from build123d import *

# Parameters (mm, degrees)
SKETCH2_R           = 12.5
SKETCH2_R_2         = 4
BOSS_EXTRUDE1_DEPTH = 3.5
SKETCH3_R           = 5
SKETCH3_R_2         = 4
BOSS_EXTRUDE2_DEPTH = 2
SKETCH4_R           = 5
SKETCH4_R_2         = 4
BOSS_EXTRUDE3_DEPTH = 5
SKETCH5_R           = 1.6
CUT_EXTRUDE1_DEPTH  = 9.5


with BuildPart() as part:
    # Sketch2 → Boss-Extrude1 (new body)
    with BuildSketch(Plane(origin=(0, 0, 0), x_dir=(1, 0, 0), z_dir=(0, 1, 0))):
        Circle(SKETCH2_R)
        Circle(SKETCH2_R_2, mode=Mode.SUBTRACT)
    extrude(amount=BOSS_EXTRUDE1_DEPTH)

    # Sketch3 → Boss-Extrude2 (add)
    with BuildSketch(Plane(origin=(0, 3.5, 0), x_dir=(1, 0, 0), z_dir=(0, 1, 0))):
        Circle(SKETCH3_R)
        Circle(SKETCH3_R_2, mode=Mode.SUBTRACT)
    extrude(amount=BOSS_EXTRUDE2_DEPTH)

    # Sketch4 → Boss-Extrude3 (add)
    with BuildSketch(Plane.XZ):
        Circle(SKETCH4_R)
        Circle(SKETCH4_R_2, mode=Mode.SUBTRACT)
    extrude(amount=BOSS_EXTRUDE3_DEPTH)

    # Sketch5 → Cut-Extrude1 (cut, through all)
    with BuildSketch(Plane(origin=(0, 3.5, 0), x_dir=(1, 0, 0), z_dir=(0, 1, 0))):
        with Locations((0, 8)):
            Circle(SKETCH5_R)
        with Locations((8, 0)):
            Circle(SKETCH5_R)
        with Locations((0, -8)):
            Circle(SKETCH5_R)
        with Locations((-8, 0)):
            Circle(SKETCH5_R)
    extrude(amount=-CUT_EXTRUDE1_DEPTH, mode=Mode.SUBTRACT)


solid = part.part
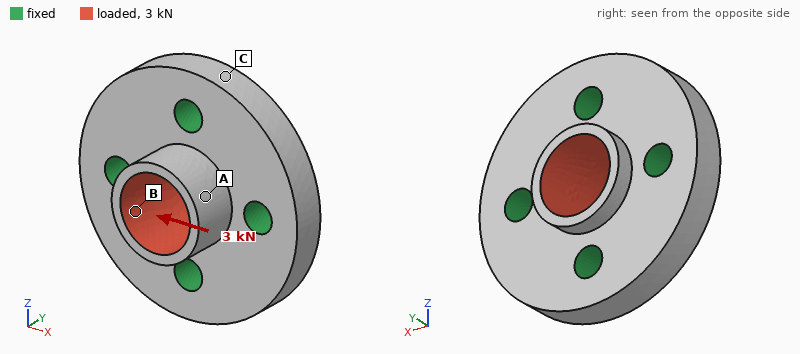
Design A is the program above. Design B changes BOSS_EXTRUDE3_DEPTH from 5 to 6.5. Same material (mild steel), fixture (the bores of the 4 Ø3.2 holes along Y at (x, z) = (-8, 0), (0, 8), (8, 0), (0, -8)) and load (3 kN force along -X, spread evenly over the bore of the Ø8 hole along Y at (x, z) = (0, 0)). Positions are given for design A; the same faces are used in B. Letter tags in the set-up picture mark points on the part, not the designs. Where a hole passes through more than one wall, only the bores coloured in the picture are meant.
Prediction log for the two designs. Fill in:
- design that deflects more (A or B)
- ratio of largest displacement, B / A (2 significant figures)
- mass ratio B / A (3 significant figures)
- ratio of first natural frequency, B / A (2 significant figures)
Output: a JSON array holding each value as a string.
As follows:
["B", "1.4", "1.03", "0.85"]
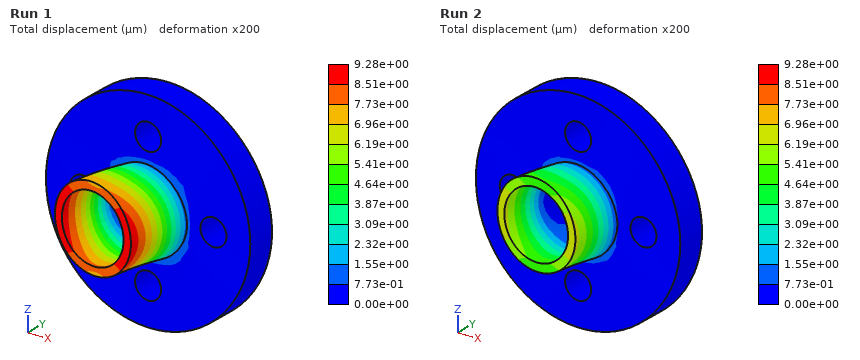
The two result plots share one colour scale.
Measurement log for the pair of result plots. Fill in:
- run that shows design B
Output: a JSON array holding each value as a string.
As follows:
["Run 1"]
